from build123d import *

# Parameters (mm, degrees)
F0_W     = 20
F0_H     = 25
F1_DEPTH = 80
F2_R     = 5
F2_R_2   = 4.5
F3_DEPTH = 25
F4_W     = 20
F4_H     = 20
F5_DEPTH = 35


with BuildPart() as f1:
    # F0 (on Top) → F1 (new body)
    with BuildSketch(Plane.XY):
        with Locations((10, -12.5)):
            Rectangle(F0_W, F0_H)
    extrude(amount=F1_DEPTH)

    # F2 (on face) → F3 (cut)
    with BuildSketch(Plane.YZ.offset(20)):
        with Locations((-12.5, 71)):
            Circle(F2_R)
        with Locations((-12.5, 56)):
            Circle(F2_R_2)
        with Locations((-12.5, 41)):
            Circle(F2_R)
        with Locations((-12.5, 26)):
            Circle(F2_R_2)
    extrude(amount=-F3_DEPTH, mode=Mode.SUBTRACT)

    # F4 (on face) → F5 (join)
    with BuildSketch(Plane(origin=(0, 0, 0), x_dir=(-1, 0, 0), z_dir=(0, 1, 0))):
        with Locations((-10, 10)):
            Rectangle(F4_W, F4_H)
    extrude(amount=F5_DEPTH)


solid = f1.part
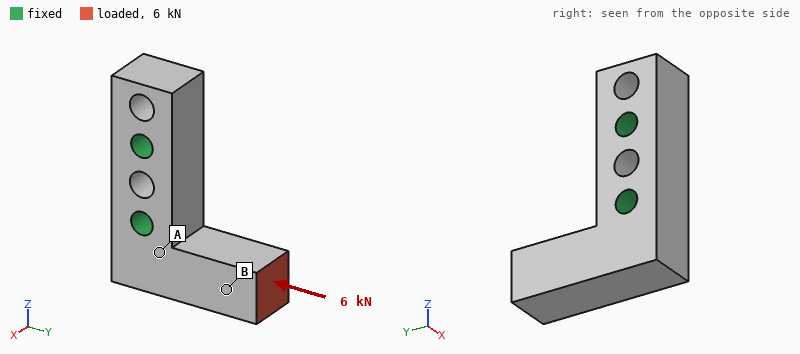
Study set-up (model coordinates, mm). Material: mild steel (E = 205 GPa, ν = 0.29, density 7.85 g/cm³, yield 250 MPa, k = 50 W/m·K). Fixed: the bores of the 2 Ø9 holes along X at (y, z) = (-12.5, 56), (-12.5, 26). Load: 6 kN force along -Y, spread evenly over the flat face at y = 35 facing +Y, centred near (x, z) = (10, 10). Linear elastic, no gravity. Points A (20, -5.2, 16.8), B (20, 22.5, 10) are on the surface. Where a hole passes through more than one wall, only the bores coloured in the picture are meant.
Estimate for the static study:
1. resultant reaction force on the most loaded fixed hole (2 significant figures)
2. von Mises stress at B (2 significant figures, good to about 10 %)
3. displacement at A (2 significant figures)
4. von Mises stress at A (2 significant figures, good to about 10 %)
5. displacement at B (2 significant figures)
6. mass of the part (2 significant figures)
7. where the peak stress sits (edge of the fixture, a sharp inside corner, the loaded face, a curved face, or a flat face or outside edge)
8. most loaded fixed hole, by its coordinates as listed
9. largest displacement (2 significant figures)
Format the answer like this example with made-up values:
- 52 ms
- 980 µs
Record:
- 6.9 kN
- 15 MPa
- 3.0 µm
- 30 MPa
- 13 µm
- 380 g
- edge of the fixture
- (-12.5, 26)
- 19 µm
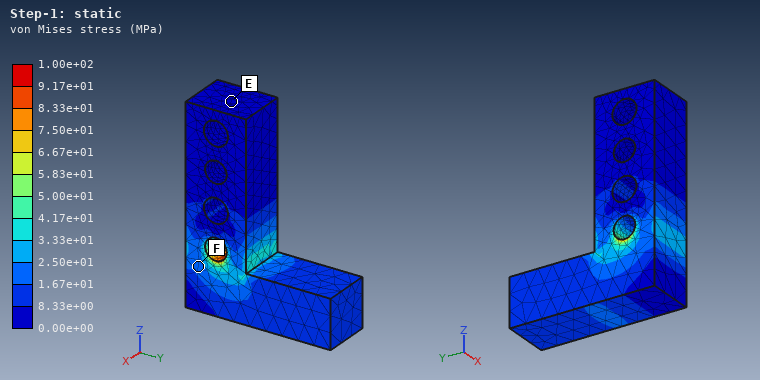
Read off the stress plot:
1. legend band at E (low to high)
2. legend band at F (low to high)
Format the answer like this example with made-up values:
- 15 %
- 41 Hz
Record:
- 0.00e+00 to 8.33e+00 MPa
- 1.67e+01 to 2.50e+01 MPa
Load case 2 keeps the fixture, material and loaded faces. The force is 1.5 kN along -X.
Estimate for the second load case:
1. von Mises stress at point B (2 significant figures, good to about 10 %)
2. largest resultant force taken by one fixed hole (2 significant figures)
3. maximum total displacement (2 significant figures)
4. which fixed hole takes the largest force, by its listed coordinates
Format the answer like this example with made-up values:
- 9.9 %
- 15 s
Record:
- 14 MPa
- 1.5 kN
- 30 µm
- (-12.5, 26)
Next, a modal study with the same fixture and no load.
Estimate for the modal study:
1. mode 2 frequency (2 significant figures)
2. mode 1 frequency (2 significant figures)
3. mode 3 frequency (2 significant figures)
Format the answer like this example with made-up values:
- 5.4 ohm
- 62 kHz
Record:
- 5600 Hz
- 5500 Hz
- 14 kHz
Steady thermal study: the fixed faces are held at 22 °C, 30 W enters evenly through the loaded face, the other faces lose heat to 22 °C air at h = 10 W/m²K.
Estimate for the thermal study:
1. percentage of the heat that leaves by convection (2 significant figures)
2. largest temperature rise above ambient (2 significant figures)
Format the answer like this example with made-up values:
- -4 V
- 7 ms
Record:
- 5.3 %
- 73 K
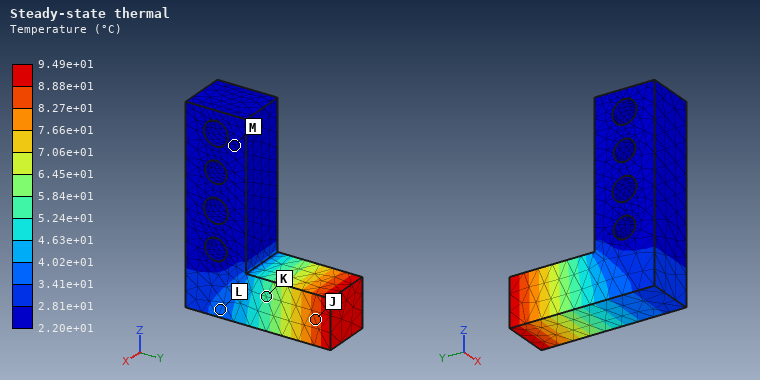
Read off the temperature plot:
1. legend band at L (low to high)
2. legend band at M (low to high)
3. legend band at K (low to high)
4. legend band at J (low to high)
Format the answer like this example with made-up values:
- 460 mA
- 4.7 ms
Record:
- 3.41e+01 to 4.02e+01 °C
- 2.20e+01 to 2.81e+01 °C
- 5.24e+01 to 5.84e+01 °C
- 8.27e+01 to 8.88e+01 °C
